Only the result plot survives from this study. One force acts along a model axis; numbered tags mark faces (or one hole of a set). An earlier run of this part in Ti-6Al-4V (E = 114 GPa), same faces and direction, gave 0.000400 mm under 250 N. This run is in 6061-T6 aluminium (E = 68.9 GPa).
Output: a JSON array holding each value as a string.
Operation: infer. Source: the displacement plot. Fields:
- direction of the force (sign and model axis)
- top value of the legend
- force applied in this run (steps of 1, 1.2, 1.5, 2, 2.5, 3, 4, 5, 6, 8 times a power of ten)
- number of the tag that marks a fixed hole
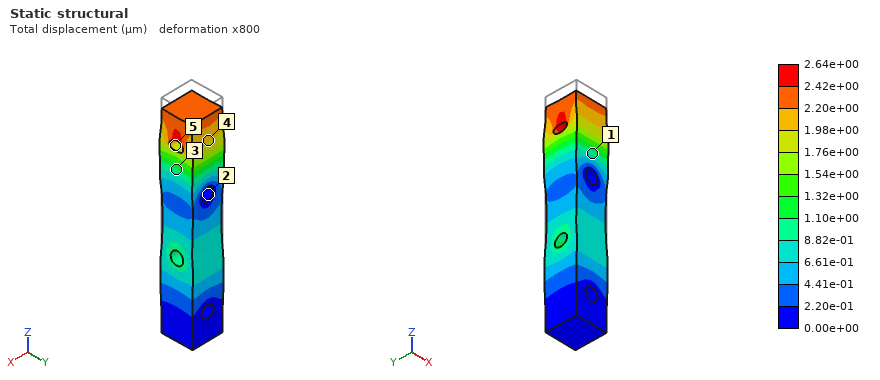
["-Z", "2.64e+00 µm", "1 kN", "2"]
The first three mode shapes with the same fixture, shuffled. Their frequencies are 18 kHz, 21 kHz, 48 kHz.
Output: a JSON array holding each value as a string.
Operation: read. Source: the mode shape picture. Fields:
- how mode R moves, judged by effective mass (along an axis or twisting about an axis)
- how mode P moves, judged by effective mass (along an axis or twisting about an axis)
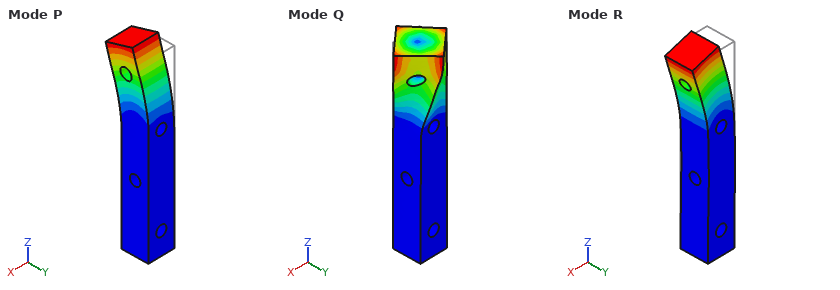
["along X", "along Y"]
